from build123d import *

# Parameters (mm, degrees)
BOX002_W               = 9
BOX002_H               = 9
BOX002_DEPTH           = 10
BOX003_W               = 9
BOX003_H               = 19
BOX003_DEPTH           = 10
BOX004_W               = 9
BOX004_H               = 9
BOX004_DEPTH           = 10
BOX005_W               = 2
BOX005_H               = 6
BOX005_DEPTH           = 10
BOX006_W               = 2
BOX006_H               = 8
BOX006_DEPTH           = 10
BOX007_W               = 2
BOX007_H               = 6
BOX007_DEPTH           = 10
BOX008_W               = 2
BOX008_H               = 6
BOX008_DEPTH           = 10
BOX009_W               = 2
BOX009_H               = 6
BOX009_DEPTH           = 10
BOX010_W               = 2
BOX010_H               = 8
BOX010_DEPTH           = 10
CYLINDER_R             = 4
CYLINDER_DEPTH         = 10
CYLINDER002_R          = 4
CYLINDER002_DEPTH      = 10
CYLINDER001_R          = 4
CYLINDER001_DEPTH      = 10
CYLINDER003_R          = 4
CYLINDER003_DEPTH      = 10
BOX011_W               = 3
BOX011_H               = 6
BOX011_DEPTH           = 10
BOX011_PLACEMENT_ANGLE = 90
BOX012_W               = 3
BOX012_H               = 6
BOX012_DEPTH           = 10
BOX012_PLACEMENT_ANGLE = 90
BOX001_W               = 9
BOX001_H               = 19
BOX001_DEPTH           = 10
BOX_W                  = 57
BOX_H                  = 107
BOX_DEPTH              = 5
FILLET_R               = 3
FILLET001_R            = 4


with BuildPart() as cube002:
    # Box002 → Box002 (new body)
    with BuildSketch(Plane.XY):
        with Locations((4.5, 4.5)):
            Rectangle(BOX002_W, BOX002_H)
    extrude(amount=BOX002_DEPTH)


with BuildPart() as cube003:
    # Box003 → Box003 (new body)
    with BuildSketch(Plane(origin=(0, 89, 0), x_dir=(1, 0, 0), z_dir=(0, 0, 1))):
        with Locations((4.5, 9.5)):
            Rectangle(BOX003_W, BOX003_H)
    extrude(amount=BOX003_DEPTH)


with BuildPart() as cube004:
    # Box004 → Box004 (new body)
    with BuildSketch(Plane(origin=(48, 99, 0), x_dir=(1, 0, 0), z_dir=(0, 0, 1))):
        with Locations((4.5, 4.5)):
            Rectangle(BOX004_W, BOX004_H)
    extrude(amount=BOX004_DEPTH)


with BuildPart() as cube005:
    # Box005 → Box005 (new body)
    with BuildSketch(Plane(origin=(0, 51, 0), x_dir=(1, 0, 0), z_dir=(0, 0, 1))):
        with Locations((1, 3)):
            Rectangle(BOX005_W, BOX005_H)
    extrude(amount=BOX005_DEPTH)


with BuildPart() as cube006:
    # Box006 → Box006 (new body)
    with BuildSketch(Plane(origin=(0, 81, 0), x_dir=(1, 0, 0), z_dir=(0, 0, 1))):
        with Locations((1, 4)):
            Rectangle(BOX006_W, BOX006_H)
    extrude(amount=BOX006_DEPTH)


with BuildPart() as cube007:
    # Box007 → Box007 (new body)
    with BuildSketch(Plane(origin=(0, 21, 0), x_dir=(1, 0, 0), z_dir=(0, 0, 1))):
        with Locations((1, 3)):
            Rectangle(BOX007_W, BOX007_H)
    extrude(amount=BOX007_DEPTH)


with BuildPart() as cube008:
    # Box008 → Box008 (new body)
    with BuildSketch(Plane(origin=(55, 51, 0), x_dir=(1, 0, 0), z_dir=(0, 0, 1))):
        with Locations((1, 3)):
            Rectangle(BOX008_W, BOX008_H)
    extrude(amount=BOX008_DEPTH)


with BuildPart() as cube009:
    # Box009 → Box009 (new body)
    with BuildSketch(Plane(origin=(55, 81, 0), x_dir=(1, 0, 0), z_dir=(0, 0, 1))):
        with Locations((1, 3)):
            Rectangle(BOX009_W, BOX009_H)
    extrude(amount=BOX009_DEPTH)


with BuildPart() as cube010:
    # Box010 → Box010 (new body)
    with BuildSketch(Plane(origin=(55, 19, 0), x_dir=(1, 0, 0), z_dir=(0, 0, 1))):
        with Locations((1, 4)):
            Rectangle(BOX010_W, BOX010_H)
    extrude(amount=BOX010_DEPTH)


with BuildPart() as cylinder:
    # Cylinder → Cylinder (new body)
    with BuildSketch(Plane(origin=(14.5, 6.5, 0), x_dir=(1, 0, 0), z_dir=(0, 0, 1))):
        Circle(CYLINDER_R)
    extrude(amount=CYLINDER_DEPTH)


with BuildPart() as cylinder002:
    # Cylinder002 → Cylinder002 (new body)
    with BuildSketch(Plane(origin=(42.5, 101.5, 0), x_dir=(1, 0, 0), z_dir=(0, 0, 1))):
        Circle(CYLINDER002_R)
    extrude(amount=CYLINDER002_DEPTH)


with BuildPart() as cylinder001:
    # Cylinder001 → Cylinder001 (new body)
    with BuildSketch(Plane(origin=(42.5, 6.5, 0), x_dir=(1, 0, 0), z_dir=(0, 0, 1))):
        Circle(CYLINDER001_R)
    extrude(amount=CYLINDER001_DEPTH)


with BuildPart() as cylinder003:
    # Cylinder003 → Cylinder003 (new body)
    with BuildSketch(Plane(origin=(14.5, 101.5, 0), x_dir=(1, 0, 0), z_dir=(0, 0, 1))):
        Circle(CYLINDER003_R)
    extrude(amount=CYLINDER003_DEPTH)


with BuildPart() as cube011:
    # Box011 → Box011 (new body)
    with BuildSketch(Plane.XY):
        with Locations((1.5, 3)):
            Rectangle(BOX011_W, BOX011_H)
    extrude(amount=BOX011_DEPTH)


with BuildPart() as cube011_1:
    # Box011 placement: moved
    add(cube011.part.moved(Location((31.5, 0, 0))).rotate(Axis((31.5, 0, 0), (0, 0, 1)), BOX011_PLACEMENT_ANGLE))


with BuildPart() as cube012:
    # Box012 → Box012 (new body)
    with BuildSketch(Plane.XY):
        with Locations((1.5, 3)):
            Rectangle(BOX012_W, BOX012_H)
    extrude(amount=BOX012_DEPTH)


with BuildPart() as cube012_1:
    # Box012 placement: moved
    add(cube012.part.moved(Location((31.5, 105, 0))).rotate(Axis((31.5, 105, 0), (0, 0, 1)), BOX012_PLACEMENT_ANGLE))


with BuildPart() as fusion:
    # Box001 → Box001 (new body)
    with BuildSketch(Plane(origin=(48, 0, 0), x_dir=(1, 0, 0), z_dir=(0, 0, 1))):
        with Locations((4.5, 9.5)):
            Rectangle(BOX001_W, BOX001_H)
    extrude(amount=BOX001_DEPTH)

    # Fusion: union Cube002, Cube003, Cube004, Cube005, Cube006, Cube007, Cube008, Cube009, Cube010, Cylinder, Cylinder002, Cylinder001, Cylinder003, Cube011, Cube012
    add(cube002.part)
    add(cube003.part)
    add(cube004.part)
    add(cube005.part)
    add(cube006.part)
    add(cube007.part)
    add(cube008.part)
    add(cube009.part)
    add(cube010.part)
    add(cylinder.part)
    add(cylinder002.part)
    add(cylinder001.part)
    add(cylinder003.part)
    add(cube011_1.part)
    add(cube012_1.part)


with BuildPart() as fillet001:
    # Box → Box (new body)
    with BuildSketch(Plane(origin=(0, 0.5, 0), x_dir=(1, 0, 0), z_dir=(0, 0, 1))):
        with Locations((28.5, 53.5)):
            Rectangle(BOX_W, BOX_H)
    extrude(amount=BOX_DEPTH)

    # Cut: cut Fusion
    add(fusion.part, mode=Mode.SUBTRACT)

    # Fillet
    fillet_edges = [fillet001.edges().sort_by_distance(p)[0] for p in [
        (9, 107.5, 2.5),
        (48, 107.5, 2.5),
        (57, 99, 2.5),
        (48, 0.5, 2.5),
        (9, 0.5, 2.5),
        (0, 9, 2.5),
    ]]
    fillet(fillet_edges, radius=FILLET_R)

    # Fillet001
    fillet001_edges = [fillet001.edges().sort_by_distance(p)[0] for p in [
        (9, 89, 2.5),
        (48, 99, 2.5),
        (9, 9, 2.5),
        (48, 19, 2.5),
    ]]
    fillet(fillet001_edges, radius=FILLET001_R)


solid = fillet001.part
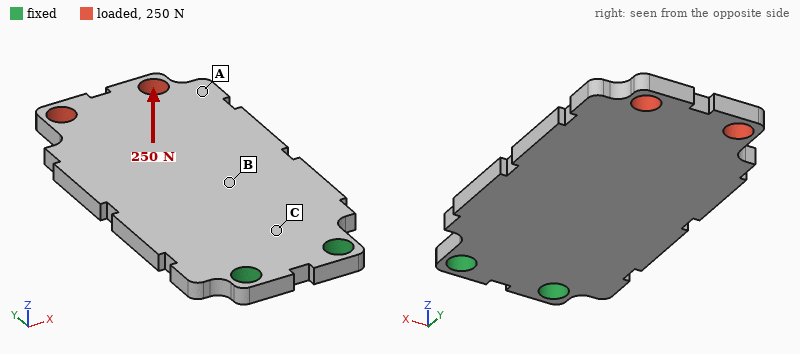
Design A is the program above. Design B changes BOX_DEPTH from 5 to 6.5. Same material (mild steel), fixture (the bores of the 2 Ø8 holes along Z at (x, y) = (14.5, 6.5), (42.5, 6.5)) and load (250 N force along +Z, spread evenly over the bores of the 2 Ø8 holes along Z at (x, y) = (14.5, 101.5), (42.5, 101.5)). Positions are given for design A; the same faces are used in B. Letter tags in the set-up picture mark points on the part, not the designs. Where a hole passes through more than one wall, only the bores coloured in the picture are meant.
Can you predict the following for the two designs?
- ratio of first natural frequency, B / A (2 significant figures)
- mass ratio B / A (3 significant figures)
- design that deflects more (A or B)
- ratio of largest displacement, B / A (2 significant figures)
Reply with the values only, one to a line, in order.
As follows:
1.3
1.30
A
0.46
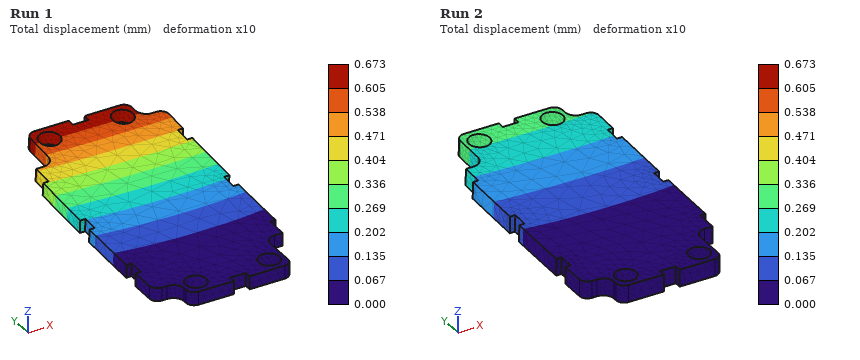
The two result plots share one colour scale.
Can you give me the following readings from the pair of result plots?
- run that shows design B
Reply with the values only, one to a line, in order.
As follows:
Run 2
